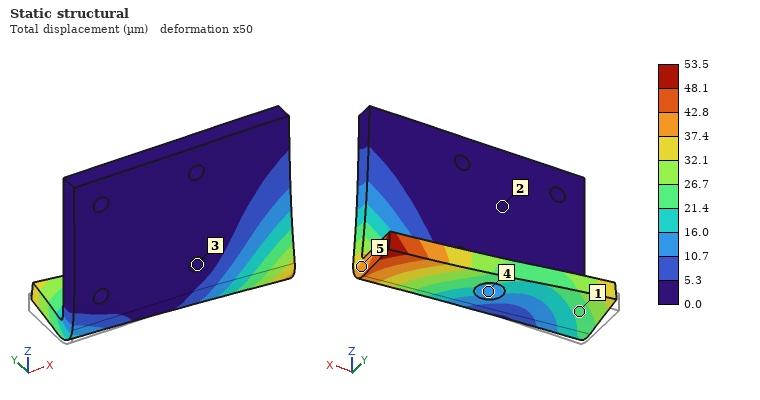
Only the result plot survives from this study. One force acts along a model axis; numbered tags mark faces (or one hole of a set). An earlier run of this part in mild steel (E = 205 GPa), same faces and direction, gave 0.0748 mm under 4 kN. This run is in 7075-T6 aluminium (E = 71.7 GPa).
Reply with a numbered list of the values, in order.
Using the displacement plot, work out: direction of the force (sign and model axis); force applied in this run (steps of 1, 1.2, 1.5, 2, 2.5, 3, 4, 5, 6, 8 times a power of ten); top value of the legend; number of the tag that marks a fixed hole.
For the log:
1. +X
2. 1 kN
3. 53.5 µm
4. 3
